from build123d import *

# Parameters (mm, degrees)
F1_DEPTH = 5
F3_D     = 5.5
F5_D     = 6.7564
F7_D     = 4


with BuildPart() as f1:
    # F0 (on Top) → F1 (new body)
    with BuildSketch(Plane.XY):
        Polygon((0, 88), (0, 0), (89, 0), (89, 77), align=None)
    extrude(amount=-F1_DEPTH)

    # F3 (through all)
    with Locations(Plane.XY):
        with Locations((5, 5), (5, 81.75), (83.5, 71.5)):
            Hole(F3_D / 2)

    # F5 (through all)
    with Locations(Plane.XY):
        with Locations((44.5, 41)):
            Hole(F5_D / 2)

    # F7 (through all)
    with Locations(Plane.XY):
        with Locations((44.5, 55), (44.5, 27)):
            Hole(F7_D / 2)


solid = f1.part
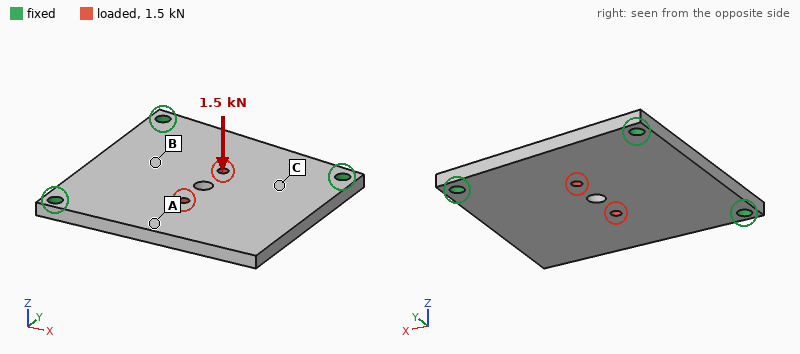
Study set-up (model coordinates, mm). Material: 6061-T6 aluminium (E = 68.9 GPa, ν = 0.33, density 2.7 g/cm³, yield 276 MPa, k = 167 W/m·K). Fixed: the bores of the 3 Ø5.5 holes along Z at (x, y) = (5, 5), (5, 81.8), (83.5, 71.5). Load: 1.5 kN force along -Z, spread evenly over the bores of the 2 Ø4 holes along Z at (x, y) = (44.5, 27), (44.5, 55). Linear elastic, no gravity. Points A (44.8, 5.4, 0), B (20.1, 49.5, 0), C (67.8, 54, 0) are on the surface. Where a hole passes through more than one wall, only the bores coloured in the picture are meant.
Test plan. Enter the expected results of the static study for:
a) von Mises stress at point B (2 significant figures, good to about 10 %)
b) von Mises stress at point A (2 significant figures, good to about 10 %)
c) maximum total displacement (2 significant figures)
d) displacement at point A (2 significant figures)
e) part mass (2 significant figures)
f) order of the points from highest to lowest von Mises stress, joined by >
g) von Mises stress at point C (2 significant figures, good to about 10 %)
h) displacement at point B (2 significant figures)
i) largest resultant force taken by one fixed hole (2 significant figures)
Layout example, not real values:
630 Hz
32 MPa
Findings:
25 MPa
45 MPa
0.36 mm
0.24 mm
97 g
A > B > C
13 MPa
0.100 mm
660 N
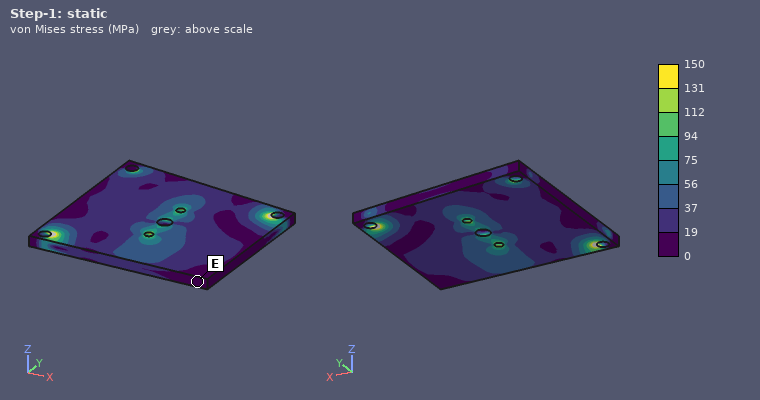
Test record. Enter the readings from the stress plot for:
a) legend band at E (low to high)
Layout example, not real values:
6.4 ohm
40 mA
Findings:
0 to 19 MPa
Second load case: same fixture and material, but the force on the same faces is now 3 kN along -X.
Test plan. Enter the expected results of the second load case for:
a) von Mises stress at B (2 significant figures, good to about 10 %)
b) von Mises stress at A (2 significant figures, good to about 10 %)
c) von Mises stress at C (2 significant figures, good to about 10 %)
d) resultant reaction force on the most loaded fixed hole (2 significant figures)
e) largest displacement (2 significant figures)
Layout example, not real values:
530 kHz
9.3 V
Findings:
4.1 MPa
5.0 MPa
6.7 MPa
1.2 kN
9.4 µm
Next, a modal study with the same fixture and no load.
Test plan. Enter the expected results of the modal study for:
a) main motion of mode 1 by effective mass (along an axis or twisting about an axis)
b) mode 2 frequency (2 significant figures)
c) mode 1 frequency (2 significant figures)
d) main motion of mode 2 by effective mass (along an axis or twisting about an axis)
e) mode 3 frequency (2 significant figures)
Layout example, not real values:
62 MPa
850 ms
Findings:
along Z
3100 Hz
1300 Hz
along Z
4500 Hz
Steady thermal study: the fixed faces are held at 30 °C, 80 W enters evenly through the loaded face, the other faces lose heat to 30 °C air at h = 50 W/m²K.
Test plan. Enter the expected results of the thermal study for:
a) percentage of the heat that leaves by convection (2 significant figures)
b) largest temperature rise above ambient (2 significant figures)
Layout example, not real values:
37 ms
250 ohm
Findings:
22 %
47 K
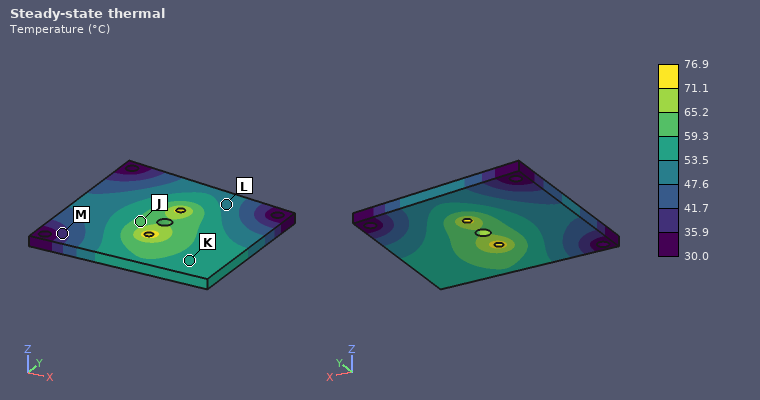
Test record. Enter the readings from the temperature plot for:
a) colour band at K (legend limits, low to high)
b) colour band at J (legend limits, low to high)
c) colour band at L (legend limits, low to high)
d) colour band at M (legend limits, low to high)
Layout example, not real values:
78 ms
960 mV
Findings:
53.5 to 59.3 °C
59.3 to 65.2 °C
47.6 to 53.5 °C
35.9 to 41.7 °C
